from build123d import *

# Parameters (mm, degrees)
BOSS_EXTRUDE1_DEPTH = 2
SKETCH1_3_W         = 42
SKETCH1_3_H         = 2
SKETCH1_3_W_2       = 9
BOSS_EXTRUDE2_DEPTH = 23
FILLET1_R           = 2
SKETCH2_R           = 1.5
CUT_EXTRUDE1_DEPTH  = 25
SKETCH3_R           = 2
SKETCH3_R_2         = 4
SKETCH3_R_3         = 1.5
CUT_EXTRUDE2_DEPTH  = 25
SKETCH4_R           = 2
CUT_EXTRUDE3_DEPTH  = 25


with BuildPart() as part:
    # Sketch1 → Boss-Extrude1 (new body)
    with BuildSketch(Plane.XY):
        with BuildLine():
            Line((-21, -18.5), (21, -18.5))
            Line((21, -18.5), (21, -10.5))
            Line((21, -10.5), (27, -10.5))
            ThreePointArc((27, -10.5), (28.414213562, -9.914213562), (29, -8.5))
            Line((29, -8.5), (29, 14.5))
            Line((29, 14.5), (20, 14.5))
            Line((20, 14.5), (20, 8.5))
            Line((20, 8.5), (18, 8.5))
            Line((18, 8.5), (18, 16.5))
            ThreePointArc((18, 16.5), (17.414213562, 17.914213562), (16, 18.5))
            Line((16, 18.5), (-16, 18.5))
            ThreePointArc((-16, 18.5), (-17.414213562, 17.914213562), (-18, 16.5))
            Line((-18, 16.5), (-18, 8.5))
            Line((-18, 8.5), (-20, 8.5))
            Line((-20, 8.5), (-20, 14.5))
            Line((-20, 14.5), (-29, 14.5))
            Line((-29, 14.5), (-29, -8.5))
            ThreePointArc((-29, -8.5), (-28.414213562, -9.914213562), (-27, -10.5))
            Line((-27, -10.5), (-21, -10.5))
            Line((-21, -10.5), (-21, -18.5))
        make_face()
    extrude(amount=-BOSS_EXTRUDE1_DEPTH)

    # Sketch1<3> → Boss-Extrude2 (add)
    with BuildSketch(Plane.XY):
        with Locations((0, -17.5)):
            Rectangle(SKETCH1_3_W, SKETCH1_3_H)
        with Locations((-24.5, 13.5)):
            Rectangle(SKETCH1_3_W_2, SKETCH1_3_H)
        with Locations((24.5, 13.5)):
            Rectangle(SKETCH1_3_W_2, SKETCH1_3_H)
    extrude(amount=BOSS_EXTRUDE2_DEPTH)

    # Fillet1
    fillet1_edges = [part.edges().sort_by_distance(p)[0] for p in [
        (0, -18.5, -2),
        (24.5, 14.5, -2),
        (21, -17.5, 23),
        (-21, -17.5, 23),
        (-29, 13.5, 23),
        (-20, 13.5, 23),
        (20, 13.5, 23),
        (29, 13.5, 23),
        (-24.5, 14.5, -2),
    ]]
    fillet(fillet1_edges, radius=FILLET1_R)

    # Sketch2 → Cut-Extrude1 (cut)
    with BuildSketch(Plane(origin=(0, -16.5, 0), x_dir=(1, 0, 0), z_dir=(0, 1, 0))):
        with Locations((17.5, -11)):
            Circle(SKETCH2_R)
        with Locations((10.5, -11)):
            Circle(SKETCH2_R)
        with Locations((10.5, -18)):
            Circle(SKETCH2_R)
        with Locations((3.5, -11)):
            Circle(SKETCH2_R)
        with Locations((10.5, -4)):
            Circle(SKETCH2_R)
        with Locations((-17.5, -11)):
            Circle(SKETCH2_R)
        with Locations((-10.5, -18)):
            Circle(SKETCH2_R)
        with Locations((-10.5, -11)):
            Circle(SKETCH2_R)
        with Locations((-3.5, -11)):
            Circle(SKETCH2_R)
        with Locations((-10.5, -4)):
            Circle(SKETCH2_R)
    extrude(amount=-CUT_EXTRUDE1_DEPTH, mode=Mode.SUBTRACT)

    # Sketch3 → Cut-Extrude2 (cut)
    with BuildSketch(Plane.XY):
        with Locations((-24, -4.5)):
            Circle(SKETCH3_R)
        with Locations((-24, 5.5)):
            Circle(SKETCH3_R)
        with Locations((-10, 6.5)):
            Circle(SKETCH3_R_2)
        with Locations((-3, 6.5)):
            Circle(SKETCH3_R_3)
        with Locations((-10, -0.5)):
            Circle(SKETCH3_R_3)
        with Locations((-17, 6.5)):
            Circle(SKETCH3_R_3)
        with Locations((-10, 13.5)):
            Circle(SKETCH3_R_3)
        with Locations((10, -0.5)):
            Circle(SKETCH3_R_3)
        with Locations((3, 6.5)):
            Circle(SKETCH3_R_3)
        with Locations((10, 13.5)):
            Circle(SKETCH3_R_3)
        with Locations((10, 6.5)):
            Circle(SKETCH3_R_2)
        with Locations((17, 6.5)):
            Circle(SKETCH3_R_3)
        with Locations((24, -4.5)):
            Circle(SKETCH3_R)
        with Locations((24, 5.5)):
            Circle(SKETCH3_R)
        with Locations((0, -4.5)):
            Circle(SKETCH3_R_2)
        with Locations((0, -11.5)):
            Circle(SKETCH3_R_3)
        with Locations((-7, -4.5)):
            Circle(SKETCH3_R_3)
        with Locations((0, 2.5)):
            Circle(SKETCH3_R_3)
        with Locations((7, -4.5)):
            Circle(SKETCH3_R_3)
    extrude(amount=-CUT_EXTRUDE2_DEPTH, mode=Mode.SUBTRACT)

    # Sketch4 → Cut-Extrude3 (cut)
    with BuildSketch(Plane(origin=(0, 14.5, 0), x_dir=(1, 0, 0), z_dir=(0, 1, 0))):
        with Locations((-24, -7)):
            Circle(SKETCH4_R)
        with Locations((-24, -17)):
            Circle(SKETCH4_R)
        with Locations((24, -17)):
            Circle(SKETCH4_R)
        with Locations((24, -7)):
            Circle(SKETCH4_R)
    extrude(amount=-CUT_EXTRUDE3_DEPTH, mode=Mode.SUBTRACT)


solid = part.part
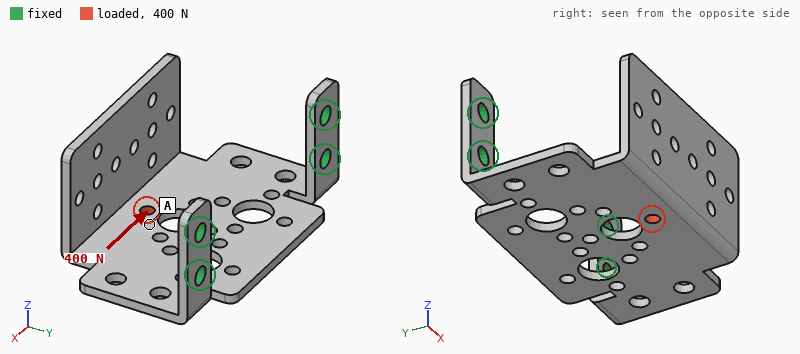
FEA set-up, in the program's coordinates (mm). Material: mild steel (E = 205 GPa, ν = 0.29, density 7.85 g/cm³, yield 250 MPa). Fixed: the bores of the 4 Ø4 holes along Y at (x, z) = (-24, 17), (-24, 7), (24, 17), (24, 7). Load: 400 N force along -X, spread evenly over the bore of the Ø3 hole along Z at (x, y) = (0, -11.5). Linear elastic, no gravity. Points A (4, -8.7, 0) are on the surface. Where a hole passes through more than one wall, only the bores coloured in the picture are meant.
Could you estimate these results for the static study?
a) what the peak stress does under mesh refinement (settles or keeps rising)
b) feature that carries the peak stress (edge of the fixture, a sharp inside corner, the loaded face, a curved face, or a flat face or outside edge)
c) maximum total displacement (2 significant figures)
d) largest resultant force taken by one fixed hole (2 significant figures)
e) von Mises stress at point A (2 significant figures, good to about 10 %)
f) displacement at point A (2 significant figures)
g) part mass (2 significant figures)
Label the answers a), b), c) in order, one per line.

a) keeps rising
b) edge of the fixture
c) 61 µm
d) 310 N
e) 19 MPa
f) 23 µm
g) 45 g
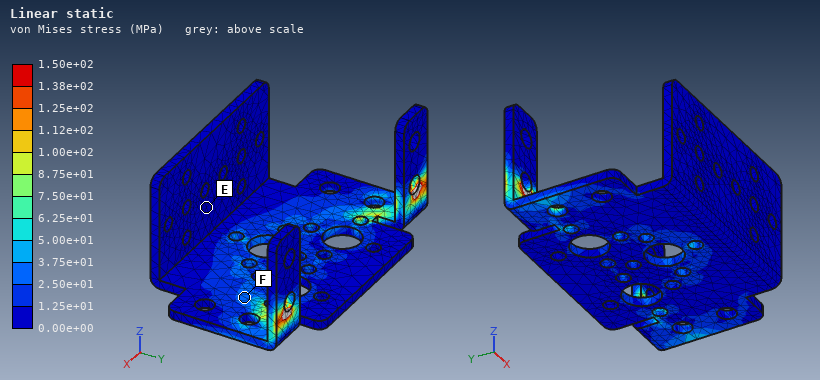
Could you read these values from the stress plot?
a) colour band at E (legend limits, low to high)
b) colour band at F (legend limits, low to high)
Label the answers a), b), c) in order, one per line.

a) 0.00e+00 to 1.25e+01 MPa
b) 2.50e+01 to 3.75e+01 MPa
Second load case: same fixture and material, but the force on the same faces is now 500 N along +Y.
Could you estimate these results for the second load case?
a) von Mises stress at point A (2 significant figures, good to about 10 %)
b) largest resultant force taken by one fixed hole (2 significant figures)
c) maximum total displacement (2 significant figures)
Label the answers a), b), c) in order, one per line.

a) 16 MPa
b) 260 N
c) 0.16 mm
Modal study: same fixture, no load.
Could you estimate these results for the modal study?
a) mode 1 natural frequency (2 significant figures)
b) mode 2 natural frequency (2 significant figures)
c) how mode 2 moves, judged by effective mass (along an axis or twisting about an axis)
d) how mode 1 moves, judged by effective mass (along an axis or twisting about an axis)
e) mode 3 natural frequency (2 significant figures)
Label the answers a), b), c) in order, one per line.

a) 410 Hz
b) 1200 Hz
c) along X
d) along Z
e) 1600 Hz
